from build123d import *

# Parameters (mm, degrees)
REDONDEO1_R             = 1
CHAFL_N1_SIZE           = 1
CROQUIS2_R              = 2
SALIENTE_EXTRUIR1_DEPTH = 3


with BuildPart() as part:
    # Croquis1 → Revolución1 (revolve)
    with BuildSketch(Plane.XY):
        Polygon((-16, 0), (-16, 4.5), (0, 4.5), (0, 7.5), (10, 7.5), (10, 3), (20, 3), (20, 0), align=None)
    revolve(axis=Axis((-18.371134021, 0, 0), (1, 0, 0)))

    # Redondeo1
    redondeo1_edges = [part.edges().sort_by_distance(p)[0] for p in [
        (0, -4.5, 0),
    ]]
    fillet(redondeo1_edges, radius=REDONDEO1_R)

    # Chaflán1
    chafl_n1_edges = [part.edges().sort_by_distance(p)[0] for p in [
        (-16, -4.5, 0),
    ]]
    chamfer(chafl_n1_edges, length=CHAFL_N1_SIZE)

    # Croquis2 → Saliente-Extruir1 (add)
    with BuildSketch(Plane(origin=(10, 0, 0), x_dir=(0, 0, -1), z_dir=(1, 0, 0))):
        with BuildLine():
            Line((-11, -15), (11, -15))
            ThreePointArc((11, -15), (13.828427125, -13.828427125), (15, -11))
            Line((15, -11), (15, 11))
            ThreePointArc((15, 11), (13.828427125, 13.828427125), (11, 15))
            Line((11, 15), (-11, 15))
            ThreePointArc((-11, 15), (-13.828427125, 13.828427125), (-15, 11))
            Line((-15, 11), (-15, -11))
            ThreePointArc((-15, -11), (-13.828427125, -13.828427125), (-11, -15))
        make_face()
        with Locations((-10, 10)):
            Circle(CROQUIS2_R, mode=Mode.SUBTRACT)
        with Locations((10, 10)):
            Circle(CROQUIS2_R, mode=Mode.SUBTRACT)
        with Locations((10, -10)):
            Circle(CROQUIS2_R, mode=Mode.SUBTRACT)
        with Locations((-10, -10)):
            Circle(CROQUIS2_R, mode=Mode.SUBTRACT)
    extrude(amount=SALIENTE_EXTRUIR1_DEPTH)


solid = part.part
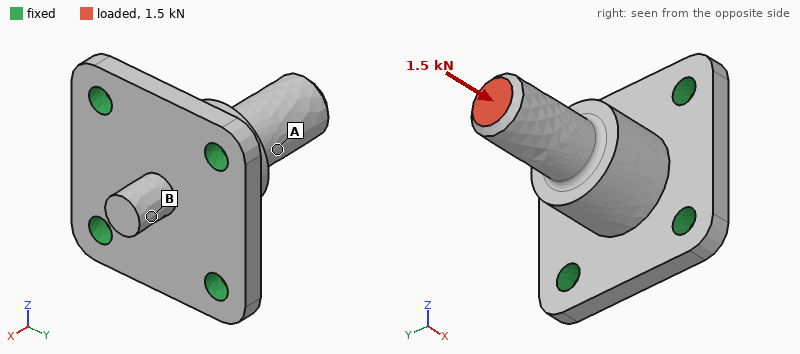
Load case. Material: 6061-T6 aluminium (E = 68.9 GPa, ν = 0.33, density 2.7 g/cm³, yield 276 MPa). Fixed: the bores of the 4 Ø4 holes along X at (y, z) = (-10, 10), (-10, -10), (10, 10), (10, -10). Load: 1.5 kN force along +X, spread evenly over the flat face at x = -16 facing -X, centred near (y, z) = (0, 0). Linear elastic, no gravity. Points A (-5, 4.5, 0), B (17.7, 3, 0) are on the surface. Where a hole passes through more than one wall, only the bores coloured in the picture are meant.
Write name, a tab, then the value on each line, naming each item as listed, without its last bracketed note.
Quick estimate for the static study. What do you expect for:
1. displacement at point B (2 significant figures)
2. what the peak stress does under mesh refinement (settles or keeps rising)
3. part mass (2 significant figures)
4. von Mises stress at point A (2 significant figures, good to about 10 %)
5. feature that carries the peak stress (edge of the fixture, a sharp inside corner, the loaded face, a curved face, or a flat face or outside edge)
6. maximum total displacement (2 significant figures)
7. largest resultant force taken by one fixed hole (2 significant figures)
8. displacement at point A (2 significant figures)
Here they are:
displacement at point B	10 µm
what the peak stress does under mesh refinement	keeps rising
part mass	15 g
von Mises stress at point A	23 MPa
feature that carries the peak stress	edge of the fixture
maximum total displacement	17 µm
largest resultant force taken by one fixed hole	390 N
displacement at point A	13 µm
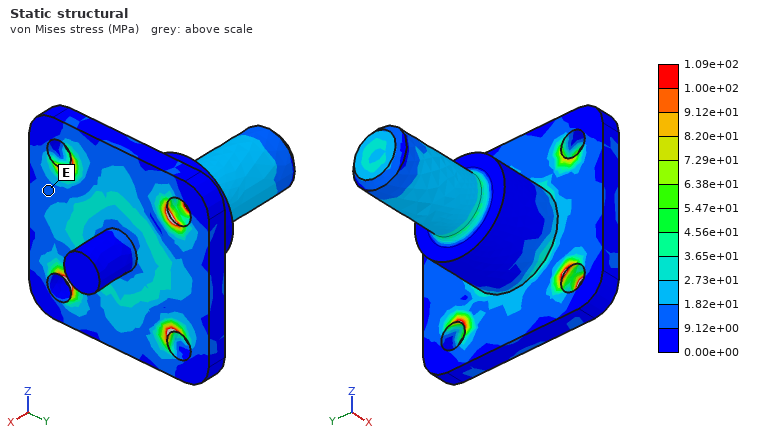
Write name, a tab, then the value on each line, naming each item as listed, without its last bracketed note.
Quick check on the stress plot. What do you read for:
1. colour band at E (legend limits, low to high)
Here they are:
colour band at E	9.12e+00 to 1.82e+01 MPa
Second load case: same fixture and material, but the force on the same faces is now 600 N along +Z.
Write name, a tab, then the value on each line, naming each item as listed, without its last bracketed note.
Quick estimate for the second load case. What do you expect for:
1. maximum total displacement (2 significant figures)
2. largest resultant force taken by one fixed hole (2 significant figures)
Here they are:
maximum total displacement	0.12 mm
largest resultant force taken by one fixed hole	530 N
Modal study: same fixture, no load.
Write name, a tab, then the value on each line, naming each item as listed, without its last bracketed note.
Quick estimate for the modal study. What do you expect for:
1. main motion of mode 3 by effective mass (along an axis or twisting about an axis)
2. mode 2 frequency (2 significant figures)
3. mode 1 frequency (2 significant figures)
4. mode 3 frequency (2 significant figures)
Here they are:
main motion of mode 3 by effective mass	along X
mode 2 frequency	10 kHz
mode 1 frequency	10 kHz
mode 3 frequency	19 kHz
